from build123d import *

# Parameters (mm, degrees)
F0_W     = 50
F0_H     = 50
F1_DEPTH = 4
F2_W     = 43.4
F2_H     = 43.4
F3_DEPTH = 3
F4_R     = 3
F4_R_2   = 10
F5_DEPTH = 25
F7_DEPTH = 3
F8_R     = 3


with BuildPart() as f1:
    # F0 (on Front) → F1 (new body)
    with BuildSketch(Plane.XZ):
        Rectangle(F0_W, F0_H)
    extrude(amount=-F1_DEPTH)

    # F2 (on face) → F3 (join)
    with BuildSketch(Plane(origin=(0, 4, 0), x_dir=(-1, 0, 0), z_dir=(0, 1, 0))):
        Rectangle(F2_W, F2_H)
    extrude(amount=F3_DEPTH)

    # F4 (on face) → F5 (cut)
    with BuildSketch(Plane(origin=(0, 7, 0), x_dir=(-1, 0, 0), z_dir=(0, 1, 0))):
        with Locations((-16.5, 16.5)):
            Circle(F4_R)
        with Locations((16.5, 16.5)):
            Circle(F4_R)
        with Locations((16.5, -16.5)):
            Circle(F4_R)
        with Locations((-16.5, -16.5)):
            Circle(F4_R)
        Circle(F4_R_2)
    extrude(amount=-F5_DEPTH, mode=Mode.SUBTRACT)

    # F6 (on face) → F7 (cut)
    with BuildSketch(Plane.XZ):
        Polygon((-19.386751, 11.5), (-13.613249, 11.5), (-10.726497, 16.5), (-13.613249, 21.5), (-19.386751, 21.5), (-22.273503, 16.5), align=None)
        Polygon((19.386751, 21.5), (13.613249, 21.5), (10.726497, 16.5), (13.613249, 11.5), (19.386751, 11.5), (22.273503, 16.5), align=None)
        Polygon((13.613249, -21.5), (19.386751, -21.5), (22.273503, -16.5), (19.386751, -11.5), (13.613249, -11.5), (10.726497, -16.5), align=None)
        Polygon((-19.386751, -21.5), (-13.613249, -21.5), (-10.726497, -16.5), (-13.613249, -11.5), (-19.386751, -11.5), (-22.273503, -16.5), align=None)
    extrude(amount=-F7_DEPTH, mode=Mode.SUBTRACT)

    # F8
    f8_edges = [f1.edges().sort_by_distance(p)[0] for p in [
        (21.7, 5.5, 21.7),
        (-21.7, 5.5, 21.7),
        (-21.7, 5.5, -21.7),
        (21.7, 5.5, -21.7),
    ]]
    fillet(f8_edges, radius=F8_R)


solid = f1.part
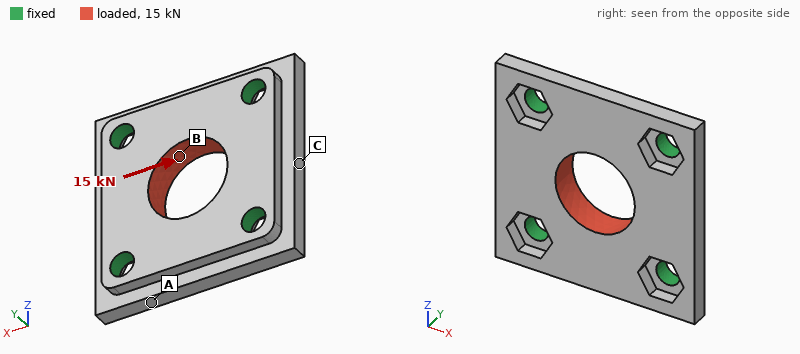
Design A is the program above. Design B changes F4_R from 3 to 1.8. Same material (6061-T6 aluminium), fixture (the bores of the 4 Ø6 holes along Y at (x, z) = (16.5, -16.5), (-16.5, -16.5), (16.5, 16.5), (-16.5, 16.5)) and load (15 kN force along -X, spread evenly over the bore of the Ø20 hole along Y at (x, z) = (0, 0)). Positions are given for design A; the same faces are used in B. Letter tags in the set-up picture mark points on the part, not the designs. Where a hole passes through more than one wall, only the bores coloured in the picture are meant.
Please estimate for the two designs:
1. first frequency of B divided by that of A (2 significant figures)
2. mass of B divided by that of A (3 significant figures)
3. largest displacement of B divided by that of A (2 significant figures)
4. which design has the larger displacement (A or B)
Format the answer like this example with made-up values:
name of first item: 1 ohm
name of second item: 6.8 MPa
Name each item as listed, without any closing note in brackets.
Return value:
first frequency of B divided by that of A: 0.82
mass of B divided by that of A: 1.02
largest displacement of B divided by that of A: 1.2
which design has the larger displacement: B
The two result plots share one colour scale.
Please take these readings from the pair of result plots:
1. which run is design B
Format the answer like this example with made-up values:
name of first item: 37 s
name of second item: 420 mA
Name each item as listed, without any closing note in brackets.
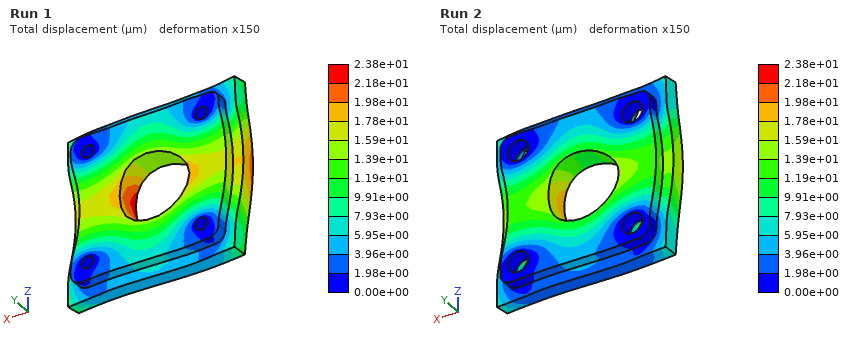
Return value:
which run is design B: Run 1
